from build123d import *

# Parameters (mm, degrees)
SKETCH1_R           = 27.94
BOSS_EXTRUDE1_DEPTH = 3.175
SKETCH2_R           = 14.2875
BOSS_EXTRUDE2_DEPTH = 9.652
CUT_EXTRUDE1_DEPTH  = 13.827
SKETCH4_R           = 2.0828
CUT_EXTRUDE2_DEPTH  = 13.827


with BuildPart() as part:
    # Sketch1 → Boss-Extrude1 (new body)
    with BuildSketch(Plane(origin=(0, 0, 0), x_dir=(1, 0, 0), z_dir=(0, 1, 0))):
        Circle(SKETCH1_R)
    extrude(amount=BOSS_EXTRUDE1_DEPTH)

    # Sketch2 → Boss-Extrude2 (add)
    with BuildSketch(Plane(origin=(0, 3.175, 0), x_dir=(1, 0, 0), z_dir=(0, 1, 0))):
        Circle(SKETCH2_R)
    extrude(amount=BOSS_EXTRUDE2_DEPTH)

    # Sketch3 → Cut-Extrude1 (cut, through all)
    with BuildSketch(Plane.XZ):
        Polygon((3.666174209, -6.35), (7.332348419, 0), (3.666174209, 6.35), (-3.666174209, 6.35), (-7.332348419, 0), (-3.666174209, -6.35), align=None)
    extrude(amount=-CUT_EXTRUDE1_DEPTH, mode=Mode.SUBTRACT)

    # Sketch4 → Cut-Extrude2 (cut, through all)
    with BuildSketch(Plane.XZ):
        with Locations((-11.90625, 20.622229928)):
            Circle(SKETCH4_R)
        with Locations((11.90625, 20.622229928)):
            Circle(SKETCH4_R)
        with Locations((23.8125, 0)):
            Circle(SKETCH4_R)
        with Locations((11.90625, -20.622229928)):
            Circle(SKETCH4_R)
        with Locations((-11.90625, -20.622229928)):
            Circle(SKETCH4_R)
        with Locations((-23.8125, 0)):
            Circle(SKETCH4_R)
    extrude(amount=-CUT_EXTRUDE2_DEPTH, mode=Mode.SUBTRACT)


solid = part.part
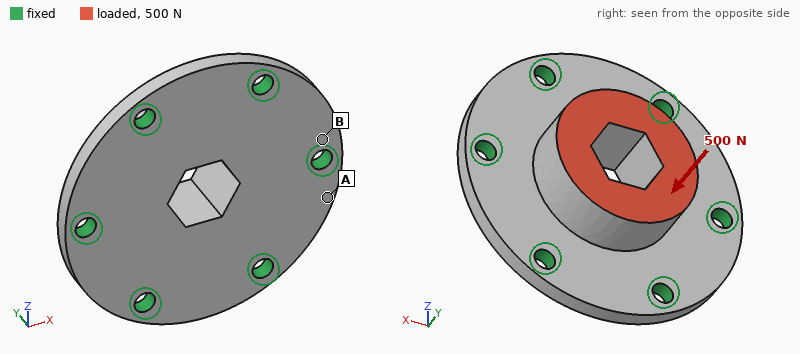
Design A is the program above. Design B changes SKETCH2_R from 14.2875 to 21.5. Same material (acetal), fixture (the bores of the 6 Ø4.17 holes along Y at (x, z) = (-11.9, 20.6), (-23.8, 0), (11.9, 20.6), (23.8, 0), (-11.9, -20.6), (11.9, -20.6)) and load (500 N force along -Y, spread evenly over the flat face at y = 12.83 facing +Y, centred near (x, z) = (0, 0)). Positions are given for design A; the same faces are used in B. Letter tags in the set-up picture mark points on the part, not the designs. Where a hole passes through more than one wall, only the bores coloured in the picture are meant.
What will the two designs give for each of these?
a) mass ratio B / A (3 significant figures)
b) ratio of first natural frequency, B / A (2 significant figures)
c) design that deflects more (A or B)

1.66
1.7
A
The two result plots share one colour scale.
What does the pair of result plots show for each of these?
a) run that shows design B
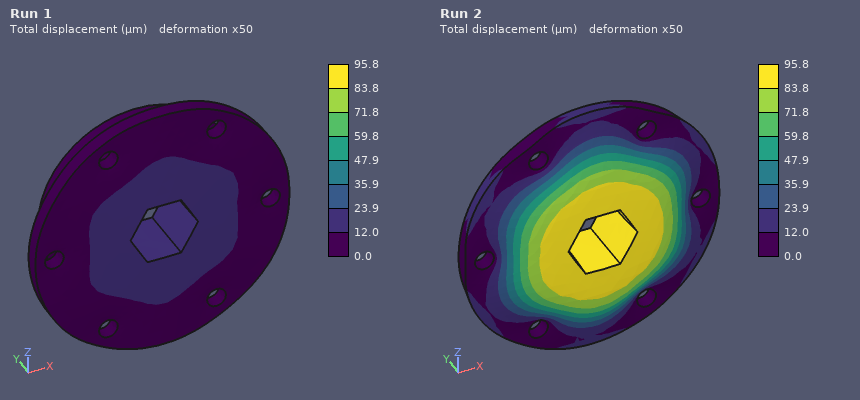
Run 1
